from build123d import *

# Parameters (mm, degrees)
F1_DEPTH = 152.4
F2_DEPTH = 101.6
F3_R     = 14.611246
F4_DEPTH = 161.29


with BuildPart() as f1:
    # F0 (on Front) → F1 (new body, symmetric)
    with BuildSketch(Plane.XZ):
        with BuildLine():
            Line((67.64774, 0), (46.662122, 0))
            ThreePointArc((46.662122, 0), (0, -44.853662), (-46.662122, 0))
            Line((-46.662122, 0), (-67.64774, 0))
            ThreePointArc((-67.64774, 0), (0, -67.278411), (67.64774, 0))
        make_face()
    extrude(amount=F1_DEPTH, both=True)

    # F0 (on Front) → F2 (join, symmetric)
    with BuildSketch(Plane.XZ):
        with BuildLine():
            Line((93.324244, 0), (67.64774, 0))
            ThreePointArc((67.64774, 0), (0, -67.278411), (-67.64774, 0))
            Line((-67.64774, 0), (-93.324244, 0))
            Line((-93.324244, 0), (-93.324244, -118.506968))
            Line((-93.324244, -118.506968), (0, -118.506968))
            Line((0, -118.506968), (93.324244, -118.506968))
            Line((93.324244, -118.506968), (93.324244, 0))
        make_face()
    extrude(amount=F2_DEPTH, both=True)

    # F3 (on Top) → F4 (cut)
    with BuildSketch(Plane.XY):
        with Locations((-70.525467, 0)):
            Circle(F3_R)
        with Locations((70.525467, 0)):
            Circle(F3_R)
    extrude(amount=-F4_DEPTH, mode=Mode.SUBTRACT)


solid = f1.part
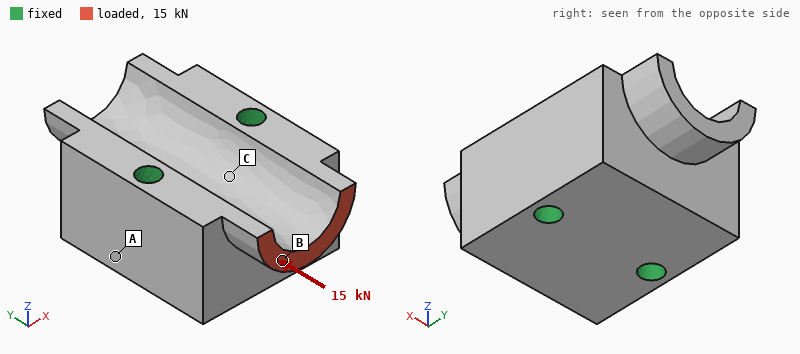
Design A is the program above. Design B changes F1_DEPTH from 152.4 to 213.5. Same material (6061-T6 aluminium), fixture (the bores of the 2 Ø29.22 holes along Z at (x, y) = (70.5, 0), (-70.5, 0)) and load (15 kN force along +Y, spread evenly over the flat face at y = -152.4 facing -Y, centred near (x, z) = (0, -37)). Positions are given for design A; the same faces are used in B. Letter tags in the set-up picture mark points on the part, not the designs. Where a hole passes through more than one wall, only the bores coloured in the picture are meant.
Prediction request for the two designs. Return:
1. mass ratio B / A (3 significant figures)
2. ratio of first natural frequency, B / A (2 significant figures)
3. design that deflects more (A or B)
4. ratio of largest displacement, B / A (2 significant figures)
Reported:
1.12
0.51
B
1.4
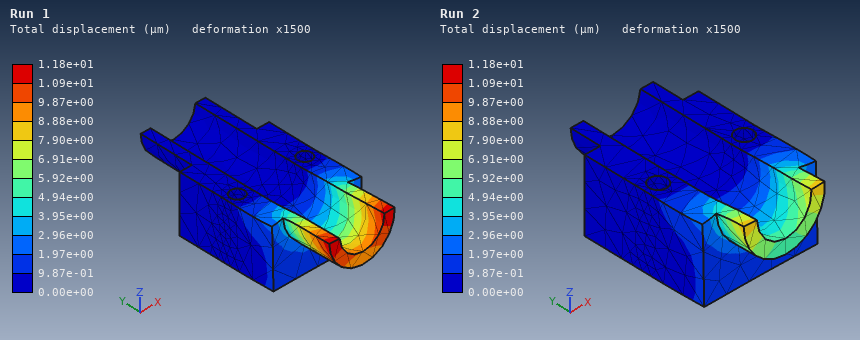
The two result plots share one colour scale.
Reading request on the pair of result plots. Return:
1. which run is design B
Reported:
Run 1
